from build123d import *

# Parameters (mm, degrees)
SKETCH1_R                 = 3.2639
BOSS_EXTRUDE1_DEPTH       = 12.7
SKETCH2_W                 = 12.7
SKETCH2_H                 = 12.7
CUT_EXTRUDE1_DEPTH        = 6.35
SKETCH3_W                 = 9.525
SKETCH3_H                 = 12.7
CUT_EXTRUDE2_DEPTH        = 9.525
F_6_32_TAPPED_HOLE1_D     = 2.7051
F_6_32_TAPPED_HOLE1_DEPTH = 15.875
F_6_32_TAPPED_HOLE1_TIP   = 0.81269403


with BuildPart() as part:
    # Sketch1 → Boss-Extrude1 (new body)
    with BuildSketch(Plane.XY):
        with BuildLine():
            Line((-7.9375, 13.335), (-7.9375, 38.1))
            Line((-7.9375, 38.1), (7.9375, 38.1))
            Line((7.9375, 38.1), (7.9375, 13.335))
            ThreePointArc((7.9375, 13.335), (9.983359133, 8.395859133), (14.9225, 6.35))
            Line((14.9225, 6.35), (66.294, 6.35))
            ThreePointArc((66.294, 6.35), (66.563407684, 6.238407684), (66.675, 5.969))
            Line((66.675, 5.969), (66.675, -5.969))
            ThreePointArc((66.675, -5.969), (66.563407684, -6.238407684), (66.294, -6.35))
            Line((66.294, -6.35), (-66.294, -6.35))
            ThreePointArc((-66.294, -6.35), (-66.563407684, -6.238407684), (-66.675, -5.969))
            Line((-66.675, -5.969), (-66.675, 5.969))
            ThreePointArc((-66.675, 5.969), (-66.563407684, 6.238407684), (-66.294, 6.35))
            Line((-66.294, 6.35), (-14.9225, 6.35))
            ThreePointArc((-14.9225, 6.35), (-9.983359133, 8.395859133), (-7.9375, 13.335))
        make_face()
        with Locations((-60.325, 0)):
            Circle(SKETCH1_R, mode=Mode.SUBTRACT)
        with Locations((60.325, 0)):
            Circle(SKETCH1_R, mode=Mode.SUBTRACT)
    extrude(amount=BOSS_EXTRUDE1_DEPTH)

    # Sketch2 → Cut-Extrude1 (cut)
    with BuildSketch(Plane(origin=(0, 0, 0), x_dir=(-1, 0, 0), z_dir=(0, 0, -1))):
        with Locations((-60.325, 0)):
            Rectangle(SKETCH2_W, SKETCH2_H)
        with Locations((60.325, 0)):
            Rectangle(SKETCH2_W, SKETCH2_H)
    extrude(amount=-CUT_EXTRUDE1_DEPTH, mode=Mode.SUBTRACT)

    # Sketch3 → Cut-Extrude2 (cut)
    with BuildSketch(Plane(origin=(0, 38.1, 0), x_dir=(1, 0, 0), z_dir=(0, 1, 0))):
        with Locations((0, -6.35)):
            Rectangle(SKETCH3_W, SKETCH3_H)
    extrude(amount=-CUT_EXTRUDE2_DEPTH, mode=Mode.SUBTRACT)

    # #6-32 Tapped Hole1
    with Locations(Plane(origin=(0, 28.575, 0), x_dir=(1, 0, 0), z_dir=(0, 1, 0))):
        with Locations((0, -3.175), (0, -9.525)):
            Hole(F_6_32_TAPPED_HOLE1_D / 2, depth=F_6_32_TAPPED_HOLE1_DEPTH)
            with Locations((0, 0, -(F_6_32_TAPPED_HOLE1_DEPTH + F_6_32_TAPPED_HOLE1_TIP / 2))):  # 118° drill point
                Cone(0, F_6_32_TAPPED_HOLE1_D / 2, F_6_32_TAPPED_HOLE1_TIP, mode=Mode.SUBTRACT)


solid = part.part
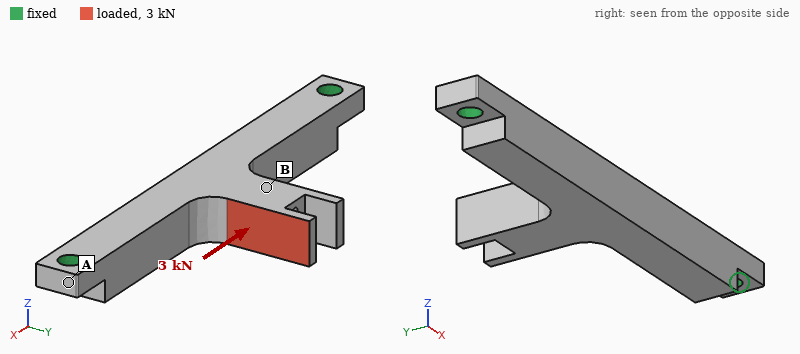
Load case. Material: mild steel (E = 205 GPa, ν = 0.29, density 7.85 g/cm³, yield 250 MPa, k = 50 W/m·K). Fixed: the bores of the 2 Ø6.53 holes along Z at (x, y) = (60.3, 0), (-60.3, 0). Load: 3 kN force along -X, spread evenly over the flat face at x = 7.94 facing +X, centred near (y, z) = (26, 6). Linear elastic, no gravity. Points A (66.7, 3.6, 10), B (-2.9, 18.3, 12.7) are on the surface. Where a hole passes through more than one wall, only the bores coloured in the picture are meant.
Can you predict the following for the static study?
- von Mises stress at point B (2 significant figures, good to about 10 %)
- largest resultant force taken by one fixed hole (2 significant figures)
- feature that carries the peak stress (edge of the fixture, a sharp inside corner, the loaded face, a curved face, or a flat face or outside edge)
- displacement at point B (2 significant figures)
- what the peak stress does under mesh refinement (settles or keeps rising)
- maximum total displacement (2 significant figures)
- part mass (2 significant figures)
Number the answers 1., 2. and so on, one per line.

1. 44 MPa
2. 1.7 kN
3. a sharp inside corner
4. 0.026 mm
5. keeps rising
6. 0.10 mm
7. 190 g
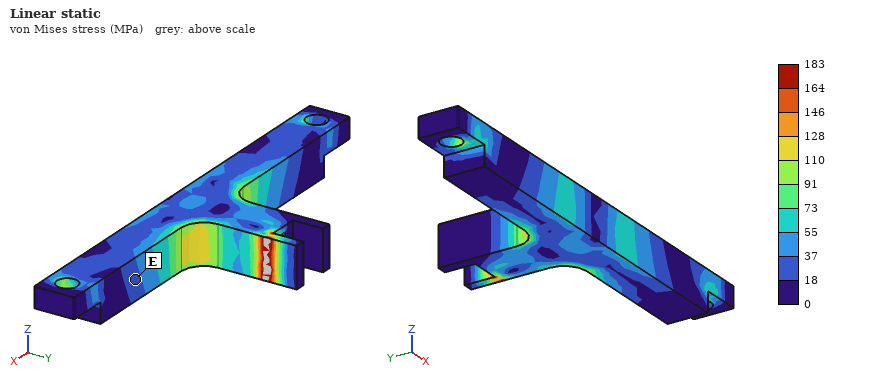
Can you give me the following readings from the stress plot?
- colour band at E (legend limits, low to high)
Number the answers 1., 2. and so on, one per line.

1. 18 to 37 MPa
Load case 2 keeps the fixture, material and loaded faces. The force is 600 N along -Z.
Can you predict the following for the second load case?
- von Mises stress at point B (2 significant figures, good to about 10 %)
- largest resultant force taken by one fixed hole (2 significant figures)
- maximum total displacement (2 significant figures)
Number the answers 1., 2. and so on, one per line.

1. 15 MPa
2. 730 N
3. 0.10 mm
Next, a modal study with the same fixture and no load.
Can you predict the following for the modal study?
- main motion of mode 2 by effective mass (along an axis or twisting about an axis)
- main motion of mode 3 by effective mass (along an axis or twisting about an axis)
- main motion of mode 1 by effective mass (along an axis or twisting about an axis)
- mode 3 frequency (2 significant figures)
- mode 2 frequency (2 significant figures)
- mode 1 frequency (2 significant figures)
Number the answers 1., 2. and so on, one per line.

1. along Y
2. along Z
3. along Z
4. 4300 Hz
5. 3100 Hz
6. 2300 Hz
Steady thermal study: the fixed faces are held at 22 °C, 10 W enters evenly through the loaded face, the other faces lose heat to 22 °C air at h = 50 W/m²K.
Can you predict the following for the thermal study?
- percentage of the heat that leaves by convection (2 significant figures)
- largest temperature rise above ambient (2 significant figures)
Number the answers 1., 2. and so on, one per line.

1. 58 %
2. 48 K
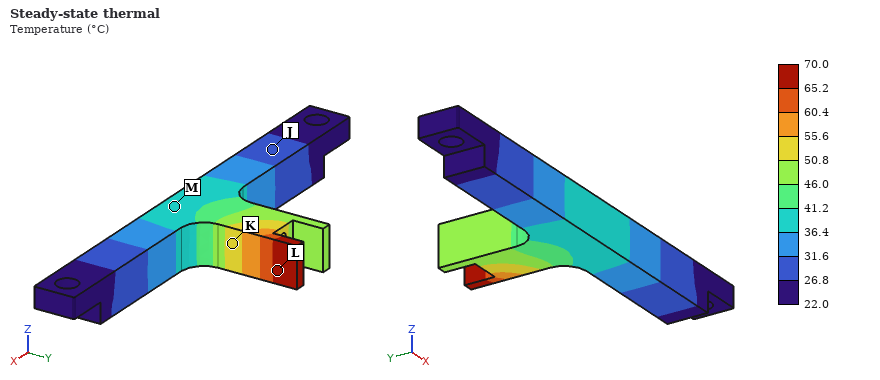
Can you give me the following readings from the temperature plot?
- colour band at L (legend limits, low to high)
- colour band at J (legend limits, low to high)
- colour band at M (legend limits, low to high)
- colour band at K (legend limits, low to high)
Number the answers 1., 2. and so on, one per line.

1. 65.2 to 70.0 °C
2. 26.8 to 31.6 °C
3. 36.4 to 41.2 °C
4. 50.8 to 55.6 °C
